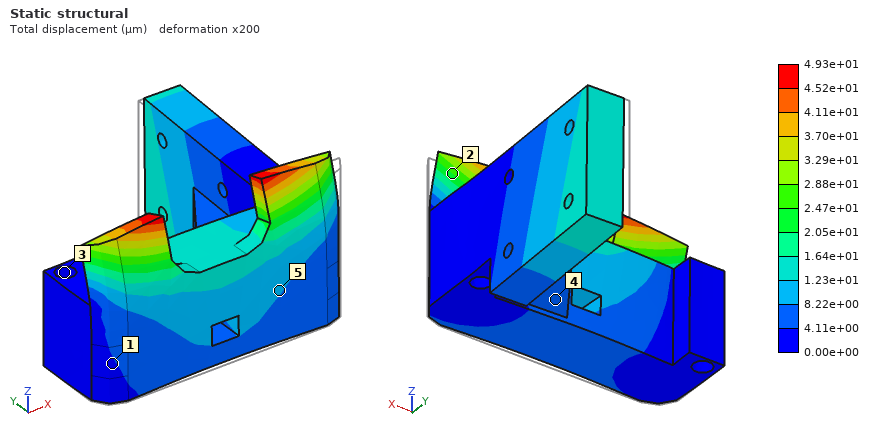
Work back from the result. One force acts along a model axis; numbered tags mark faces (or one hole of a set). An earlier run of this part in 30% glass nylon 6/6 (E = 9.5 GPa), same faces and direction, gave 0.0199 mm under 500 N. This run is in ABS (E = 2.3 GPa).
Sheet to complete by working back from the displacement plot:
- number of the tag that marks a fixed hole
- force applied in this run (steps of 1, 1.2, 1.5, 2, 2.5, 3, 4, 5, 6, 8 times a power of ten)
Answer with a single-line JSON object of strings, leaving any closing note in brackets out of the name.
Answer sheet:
{"number of the tag that marks a fixed hole": "3", "force applied in this run": "300 N"}
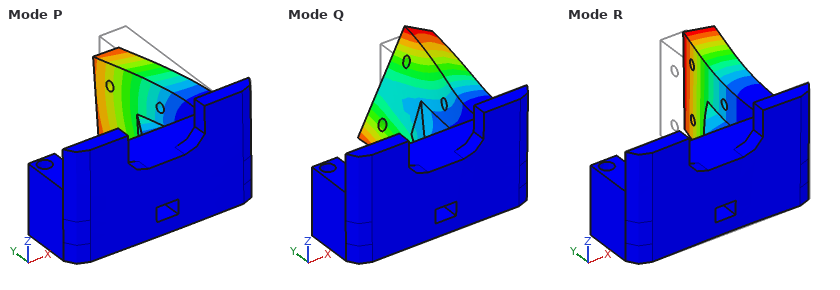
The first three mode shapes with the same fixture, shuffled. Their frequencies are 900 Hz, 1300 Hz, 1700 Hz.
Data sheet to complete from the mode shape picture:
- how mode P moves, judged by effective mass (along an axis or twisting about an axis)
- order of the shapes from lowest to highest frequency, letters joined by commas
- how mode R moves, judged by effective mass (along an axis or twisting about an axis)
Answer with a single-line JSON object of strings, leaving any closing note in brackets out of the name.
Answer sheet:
{"how mode P moves, judged by effective mass": "along Z", "order of the shapes from lowest to highest frequency, letters joined by commas": "R, P, Q", "how mode R moves, judged by effective mass": "along X"}
